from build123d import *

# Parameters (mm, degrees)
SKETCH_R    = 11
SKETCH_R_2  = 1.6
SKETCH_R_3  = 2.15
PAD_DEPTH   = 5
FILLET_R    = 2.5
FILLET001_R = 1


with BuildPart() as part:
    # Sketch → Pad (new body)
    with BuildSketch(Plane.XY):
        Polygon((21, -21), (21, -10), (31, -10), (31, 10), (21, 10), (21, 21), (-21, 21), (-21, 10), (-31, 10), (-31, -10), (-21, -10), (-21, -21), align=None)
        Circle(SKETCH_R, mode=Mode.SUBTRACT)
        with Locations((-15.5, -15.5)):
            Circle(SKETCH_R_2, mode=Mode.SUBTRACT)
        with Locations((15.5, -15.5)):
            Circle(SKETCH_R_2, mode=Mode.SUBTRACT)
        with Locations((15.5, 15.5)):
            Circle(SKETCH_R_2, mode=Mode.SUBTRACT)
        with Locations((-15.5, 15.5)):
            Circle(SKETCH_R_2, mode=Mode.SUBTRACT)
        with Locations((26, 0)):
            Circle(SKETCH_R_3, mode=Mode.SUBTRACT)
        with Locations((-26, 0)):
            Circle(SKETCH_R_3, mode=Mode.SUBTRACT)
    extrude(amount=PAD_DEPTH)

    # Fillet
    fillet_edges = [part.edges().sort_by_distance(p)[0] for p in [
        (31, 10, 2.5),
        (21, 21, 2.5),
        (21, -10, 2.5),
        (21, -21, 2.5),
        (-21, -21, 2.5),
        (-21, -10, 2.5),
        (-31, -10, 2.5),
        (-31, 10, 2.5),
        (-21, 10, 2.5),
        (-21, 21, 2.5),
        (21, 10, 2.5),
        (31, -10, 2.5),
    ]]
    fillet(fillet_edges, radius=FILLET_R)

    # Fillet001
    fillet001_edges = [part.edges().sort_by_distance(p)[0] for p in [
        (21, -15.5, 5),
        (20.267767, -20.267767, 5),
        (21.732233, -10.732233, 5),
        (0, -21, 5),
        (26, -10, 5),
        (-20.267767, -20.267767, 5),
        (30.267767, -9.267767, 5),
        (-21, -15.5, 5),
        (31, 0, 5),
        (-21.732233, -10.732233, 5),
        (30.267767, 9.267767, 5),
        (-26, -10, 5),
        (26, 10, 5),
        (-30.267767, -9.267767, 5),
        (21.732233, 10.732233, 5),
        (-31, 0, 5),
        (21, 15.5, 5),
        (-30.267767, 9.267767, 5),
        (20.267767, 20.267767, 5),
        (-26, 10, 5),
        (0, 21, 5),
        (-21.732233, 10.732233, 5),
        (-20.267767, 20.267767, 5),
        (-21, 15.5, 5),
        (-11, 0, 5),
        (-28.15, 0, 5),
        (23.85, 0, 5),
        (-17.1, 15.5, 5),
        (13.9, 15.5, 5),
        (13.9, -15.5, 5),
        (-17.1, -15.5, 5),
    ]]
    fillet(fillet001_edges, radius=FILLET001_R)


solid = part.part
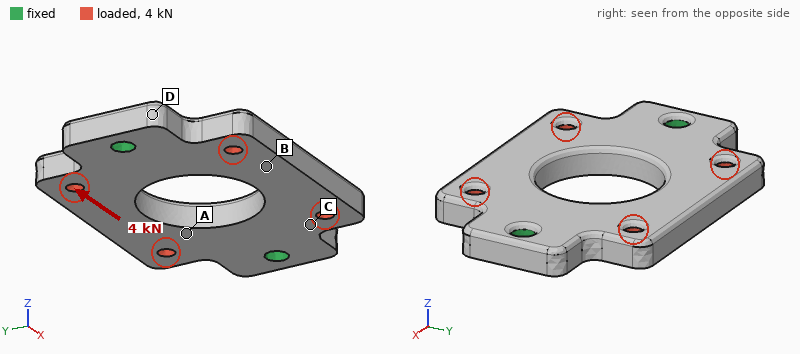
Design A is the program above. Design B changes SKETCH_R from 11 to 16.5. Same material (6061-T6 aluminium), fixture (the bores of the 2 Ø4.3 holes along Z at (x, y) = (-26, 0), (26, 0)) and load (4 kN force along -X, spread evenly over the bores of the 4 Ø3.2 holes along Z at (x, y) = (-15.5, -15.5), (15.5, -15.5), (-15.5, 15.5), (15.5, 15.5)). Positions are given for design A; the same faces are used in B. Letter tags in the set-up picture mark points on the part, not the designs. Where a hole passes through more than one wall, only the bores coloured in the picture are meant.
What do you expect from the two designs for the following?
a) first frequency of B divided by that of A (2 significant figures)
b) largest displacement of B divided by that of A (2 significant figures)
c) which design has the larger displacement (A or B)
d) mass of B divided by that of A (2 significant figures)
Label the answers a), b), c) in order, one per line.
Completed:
a) 1.0
b) 2.4
c) B
d) 0.72
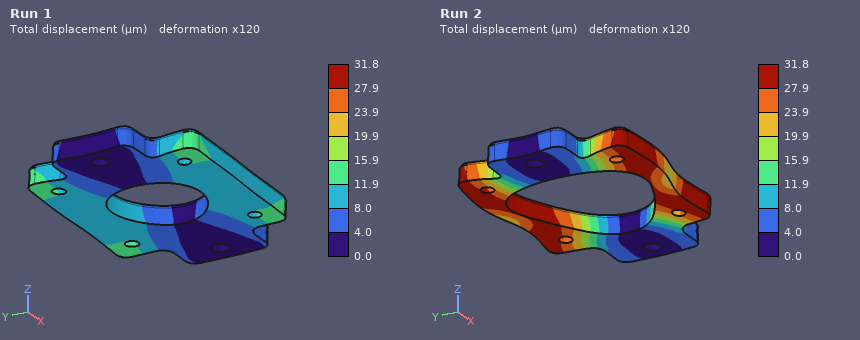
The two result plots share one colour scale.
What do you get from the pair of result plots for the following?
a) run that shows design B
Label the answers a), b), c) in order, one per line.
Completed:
a) Run 2
